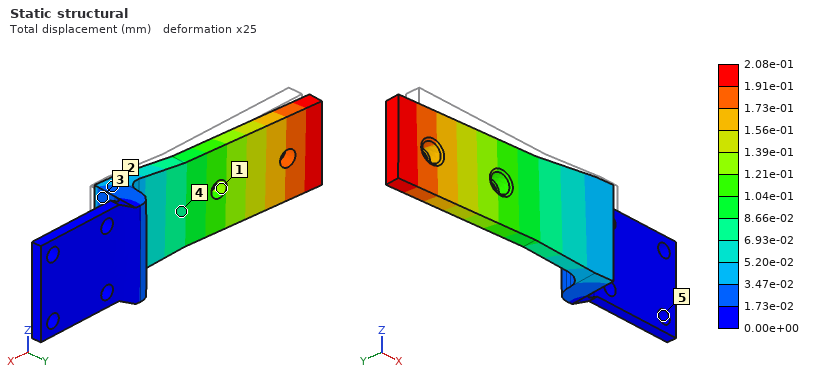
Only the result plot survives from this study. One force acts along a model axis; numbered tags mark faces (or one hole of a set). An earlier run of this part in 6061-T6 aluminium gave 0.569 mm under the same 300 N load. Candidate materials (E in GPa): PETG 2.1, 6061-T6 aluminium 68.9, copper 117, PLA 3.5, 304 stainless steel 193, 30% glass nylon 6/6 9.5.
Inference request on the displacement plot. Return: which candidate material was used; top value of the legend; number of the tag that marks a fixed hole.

304 stainless steel
2.08e-01 mm
5
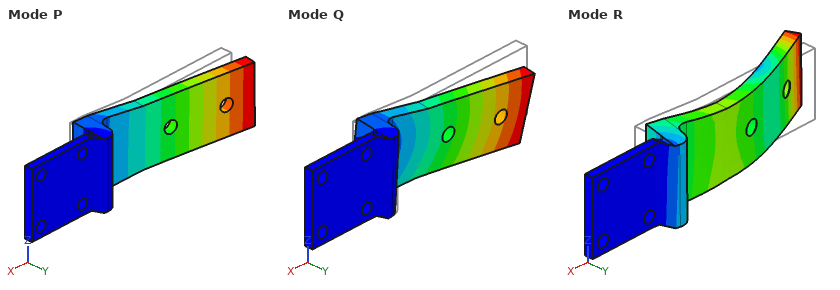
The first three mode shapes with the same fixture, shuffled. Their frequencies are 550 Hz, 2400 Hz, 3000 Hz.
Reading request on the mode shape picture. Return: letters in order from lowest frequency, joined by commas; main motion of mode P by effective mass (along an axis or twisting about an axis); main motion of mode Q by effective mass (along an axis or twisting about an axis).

P, Q, R
along Y
along Z
